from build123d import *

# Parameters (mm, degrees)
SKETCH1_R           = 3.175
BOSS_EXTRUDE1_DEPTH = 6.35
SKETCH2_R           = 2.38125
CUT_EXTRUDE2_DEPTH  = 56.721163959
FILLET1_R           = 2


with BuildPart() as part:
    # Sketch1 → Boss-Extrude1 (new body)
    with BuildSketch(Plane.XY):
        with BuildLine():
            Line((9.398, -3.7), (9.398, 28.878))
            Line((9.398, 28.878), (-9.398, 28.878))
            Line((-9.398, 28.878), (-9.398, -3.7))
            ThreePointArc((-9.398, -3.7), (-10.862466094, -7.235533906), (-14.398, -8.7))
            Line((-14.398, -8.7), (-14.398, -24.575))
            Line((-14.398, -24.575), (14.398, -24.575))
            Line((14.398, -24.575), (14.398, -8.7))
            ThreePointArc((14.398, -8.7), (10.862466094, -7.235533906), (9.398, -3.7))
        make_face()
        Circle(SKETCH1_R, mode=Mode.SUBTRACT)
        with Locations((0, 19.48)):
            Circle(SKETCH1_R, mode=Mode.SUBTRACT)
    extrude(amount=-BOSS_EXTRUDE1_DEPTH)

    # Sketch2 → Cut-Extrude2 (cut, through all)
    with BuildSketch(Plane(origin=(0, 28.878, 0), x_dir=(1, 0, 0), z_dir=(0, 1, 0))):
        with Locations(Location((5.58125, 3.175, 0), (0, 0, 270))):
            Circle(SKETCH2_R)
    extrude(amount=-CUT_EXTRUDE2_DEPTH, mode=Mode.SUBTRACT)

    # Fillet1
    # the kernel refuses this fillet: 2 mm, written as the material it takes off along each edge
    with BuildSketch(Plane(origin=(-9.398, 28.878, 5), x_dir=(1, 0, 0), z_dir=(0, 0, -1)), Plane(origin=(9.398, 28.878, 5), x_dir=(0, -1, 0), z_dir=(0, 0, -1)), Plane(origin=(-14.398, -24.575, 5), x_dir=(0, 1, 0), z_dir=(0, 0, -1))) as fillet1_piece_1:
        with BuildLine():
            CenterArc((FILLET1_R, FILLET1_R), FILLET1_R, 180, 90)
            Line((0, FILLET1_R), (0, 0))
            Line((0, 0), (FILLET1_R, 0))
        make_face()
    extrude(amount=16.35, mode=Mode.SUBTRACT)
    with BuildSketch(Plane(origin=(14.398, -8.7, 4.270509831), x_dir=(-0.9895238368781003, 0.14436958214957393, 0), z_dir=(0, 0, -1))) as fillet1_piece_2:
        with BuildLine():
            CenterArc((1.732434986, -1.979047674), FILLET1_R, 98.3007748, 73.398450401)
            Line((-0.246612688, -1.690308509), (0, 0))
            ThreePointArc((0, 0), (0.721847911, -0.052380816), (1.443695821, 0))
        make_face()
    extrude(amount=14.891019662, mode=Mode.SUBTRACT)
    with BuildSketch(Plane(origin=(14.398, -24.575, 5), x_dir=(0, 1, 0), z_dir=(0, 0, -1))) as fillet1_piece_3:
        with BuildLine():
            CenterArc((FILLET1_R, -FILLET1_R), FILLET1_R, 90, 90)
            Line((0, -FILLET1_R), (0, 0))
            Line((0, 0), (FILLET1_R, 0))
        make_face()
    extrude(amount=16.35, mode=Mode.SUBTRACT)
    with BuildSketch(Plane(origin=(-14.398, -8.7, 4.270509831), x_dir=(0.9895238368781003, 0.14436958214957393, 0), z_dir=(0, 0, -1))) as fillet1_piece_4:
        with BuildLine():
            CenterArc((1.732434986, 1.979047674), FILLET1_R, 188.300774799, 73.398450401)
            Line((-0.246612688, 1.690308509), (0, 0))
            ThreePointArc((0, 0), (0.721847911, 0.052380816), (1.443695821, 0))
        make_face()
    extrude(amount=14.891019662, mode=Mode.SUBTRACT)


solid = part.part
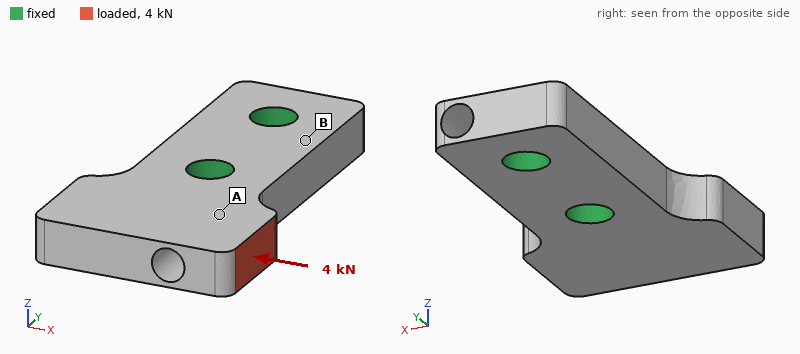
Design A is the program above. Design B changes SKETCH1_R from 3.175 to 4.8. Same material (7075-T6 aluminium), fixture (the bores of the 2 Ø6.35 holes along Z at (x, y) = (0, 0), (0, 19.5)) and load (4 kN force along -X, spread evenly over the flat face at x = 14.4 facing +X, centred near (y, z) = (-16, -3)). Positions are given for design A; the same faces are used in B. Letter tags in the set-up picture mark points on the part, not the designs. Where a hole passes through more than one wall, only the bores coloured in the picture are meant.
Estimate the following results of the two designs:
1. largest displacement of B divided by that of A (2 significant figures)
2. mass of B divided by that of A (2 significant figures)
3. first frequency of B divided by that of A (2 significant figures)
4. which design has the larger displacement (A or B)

0.74
0.92
1.2
A
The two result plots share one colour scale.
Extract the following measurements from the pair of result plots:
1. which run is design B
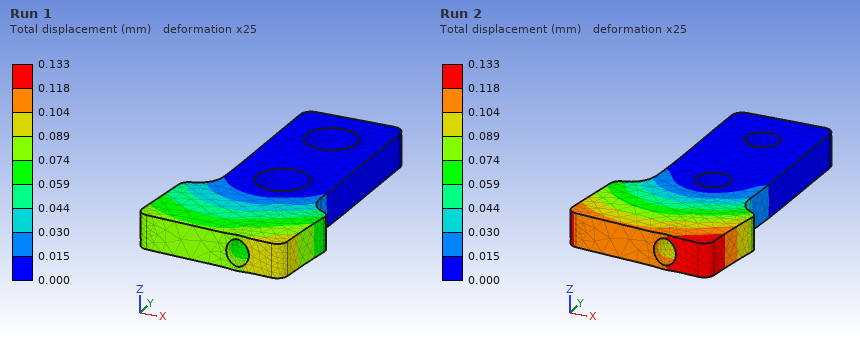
Run 1
